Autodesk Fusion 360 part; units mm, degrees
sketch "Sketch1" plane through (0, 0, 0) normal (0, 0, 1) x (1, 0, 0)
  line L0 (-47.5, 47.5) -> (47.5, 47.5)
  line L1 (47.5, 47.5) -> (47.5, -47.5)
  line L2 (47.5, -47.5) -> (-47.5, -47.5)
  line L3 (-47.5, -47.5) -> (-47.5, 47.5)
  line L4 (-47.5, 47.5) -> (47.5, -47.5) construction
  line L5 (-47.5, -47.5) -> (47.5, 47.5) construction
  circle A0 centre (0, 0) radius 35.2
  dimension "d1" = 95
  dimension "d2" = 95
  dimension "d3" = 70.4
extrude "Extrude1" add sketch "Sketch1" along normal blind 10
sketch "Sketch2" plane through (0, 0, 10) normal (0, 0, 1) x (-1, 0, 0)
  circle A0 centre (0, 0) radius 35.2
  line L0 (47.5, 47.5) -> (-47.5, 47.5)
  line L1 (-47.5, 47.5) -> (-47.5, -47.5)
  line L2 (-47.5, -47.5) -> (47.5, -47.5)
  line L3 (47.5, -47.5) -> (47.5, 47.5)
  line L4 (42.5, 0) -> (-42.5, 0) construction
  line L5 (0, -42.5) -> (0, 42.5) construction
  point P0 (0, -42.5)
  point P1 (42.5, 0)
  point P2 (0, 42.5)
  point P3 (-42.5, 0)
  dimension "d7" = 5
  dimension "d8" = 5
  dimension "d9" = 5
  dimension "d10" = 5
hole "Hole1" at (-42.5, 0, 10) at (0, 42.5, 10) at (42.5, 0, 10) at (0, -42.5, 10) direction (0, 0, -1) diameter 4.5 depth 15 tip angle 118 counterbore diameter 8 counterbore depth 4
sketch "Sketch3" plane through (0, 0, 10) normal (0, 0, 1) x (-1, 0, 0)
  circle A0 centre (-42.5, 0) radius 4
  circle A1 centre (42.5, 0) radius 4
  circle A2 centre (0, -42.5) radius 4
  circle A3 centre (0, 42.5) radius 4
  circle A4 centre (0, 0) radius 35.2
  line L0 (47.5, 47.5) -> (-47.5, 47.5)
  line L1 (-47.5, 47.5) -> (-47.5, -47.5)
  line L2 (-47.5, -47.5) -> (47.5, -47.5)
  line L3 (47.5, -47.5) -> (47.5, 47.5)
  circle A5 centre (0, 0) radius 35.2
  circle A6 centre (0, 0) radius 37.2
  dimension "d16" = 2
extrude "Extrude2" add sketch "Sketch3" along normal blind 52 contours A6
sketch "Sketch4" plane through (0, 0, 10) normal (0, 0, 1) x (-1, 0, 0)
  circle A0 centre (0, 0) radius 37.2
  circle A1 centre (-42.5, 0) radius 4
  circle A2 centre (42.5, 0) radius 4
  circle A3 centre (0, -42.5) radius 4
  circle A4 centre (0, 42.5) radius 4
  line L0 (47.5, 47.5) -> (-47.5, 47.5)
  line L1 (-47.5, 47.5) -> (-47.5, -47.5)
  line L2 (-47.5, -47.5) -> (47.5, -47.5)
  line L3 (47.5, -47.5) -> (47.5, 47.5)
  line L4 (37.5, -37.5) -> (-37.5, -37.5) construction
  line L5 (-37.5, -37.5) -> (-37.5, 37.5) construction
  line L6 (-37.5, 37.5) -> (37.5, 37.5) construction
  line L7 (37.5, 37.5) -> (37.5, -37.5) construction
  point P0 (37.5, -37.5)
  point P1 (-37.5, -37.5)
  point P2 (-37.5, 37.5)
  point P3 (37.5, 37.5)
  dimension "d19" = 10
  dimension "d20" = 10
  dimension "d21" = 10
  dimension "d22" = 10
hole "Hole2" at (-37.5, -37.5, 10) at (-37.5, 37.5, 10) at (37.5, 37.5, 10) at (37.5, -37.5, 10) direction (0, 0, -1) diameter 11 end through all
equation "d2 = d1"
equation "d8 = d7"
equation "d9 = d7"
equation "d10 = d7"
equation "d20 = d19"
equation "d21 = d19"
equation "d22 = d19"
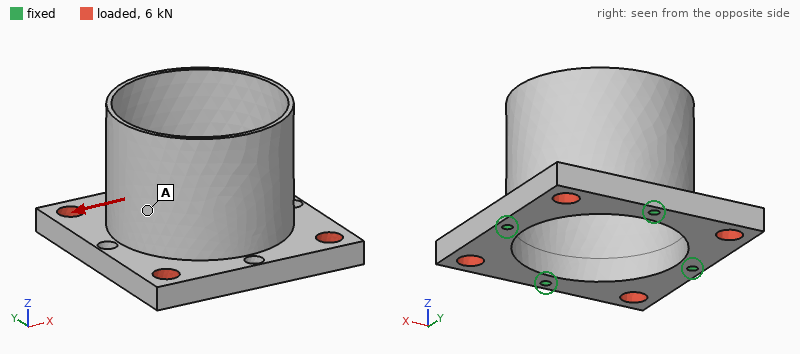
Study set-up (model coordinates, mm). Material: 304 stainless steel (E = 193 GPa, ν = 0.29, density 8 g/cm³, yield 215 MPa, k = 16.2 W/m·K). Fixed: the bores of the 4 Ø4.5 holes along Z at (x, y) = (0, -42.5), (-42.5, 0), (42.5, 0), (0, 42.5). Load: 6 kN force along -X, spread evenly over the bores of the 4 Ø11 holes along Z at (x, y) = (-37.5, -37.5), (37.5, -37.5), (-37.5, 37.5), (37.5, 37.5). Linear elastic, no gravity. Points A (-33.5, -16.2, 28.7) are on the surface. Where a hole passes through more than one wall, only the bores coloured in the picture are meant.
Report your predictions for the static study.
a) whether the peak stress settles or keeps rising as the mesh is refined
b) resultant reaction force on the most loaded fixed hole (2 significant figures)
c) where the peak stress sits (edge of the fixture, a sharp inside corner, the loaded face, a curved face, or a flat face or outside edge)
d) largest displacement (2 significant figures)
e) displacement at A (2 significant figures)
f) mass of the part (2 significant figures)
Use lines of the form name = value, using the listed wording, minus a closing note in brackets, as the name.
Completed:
whether the peak stress settles or keeps rising as the mesh is refined = keeps rising
resultant reaction force on the most loaded fixed hole = 2.7 kN
where the peak stress sits = edge of the fixture
largest displacement = 3.3 µm
displacement at A = 0.89 µm
mass of the part = 560 g
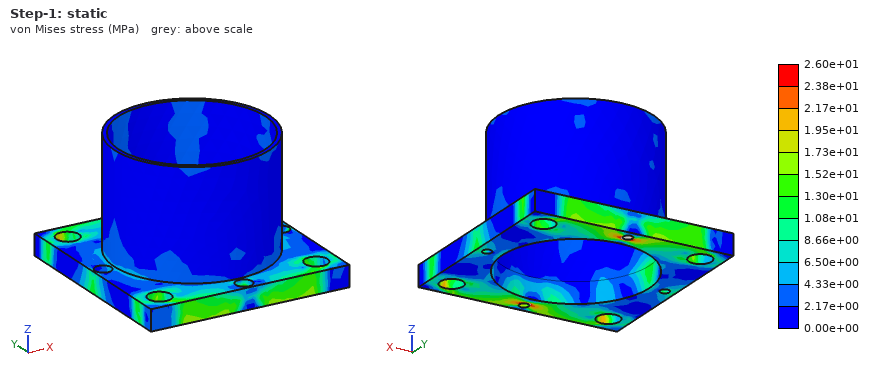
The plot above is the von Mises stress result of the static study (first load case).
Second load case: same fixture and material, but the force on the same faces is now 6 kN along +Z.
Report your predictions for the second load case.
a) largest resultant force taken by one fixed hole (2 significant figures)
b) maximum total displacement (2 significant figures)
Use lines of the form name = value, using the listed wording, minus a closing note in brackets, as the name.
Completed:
largest resultant force taken by one fixed hole = 1.5 kN
maximum total displacement = 52 µm
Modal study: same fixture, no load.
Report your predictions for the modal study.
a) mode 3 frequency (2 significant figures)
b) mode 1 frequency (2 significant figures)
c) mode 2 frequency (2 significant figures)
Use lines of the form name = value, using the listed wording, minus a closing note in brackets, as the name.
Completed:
mode 3 frequency = 3500 Hz
mode 1 frequency = 2400 Hz
mode 2 frequency = 3500 Hz
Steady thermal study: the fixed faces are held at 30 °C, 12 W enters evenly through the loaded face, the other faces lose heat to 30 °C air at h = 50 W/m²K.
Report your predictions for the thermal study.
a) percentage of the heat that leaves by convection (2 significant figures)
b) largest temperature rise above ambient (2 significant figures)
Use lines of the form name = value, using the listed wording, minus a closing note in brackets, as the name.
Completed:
percentage of the heat that leaves by convection = 61 %
largest temperature rise above ambient = 16 K
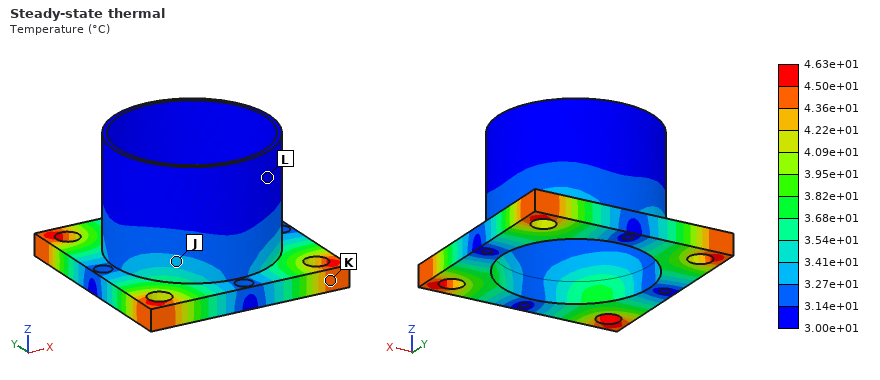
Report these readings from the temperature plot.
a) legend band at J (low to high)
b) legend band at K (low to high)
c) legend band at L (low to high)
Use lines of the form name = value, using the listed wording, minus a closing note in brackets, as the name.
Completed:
legend band at J = 3.27e+01 to 3.41e+01 °C
legend band at K = 4.36e+01 to 4.50e+01 °C
legend band at L = 3.00e+01 to 3.14e+01 °C
